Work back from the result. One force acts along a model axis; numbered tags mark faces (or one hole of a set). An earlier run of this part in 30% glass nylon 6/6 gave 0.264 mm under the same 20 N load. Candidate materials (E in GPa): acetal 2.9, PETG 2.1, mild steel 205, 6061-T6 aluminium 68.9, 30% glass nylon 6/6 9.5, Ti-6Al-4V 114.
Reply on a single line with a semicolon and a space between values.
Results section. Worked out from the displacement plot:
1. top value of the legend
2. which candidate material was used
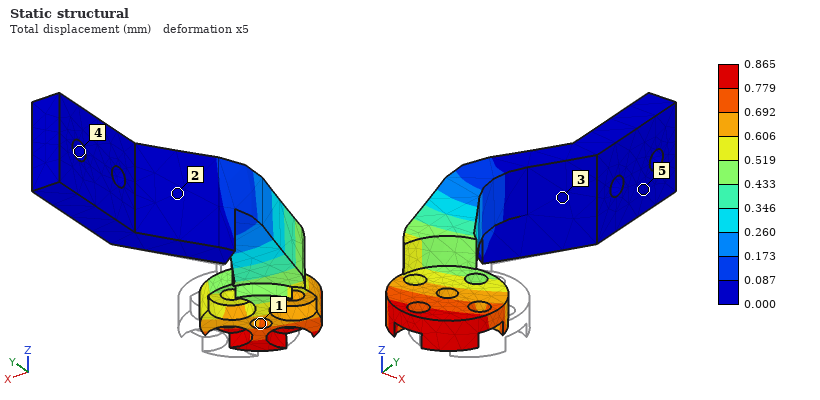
0.865 mm; acetal
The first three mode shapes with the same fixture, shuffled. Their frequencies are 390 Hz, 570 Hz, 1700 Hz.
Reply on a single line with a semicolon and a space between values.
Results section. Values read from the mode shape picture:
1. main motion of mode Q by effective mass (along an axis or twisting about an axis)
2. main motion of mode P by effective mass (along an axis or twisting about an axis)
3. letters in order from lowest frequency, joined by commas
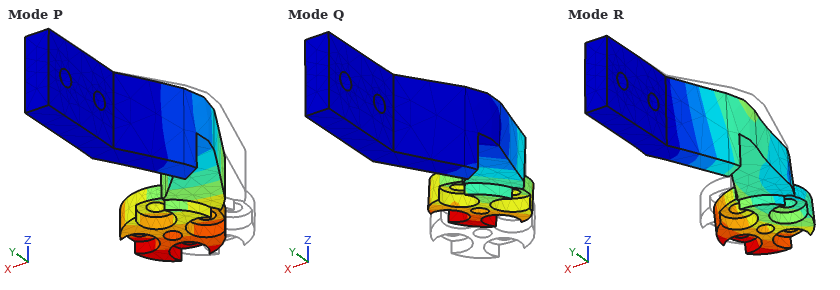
along Z; along X; P, Q, R
